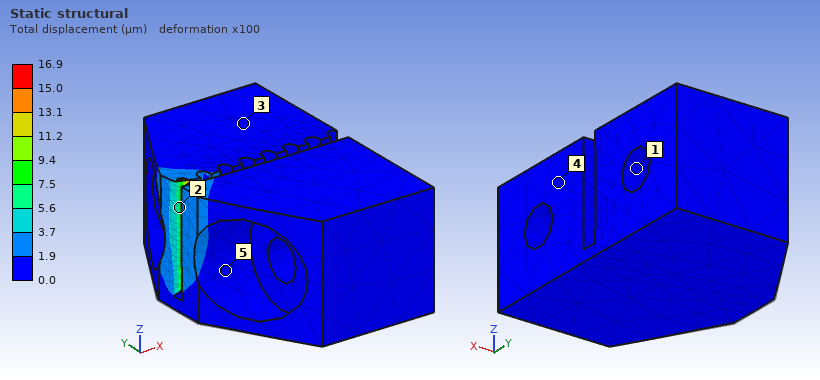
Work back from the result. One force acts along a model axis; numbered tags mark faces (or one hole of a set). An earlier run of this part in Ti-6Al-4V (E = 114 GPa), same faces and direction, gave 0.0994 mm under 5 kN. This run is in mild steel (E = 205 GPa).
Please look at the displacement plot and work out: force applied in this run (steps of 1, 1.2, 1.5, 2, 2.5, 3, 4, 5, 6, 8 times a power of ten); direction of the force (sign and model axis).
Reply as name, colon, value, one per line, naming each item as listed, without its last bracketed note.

force applied in this run: 1.5 kN
direction of the force: +X
